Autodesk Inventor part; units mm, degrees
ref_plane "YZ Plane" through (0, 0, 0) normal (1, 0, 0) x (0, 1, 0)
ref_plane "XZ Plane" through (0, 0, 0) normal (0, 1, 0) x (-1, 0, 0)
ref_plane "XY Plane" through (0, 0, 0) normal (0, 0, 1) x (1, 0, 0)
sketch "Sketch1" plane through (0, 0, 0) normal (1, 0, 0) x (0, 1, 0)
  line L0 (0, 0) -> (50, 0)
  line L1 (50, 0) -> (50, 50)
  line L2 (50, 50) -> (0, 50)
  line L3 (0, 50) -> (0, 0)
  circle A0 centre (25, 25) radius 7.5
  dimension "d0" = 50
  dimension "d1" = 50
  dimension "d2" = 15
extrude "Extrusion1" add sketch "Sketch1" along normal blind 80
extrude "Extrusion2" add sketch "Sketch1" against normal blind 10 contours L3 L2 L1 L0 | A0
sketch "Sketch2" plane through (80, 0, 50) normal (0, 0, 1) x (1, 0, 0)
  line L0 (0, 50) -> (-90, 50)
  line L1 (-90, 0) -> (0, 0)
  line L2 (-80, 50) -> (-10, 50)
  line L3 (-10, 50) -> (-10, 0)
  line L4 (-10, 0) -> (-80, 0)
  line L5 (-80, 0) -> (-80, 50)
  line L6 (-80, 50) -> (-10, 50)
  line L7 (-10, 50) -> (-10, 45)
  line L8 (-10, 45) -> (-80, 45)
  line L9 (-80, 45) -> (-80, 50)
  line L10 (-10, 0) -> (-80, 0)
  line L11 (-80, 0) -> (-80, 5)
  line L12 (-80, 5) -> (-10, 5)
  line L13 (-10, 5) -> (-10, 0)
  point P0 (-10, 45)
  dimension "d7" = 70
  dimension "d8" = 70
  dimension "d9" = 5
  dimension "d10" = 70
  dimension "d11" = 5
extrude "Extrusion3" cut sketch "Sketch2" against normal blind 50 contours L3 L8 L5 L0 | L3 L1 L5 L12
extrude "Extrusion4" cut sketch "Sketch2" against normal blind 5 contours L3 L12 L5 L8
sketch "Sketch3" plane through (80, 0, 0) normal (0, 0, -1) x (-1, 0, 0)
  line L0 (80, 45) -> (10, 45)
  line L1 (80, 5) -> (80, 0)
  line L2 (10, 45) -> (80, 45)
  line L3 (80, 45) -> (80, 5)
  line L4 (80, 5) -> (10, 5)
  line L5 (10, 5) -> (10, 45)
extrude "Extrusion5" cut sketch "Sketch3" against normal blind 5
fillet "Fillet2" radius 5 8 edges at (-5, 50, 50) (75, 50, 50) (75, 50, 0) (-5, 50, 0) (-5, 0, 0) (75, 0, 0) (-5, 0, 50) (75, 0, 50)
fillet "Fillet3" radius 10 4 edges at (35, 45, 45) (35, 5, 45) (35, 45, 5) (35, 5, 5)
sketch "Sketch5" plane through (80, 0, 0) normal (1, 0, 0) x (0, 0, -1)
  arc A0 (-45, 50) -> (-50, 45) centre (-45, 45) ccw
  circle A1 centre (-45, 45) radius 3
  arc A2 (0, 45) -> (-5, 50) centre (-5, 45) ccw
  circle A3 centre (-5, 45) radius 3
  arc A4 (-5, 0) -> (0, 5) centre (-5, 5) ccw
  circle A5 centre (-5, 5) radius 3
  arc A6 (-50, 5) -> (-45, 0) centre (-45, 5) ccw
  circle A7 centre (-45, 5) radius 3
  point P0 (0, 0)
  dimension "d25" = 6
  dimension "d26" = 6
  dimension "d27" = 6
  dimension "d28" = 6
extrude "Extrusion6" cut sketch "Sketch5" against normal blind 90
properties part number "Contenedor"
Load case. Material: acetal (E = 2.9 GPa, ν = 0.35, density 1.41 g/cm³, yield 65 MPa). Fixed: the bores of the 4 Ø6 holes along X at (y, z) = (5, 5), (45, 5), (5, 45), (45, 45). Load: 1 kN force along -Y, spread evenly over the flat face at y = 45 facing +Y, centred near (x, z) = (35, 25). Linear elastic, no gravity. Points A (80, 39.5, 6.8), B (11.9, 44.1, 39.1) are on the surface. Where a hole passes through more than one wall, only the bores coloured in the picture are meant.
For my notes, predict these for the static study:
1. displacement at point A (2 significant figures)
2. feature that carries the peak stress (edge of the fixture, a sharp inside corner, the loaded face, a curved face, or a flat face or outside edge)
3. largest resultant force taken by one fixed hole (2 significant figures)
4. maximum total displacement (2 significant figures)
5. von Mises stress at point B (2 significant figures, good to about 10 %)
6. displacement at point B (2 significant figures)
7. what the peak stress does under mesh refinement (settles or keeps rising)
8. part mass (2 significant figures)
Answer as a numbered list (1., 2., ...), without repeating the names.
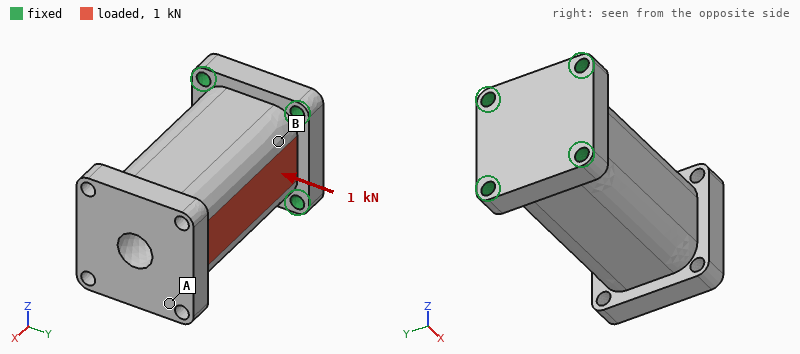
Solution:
1. 0.27 mm
2. edge of the fixture
3. 610 N
4. 0.28 mm
5. 2.8 MPa
6. 0.063 mm
7. keeps rising
8. 200 g
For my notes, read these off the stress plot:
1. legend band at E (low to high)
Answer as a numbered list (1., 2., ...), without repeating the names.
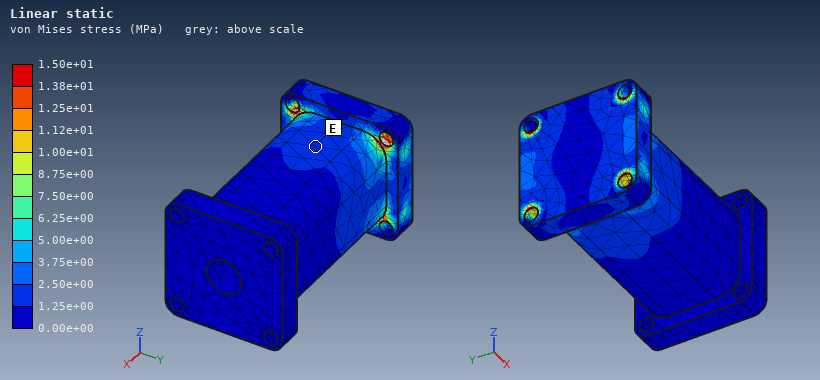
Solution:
1. 1.25e+00 to 2.50e+00 MPa
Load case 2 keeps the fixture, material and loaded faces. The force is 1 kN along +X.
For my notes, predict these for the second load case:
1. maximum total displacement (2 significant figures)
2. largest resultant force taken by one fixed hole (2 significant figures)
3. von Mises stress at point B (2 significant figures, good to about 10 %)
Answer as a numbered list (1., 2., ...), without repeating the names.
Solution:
1. 0.17 mm
2. 540 N
3. 2.8 MPa
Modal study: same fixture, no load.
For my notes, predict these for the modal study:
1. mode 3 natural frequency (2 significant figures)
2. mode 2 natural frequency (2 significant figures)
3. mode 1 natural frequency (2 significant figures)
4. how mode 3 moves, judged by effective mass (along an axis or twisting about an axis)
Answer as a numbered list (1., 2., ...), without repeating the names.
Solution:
1. 2100 Hz
2. 790 Hz
3. 790 Hz
4. twisting about X
